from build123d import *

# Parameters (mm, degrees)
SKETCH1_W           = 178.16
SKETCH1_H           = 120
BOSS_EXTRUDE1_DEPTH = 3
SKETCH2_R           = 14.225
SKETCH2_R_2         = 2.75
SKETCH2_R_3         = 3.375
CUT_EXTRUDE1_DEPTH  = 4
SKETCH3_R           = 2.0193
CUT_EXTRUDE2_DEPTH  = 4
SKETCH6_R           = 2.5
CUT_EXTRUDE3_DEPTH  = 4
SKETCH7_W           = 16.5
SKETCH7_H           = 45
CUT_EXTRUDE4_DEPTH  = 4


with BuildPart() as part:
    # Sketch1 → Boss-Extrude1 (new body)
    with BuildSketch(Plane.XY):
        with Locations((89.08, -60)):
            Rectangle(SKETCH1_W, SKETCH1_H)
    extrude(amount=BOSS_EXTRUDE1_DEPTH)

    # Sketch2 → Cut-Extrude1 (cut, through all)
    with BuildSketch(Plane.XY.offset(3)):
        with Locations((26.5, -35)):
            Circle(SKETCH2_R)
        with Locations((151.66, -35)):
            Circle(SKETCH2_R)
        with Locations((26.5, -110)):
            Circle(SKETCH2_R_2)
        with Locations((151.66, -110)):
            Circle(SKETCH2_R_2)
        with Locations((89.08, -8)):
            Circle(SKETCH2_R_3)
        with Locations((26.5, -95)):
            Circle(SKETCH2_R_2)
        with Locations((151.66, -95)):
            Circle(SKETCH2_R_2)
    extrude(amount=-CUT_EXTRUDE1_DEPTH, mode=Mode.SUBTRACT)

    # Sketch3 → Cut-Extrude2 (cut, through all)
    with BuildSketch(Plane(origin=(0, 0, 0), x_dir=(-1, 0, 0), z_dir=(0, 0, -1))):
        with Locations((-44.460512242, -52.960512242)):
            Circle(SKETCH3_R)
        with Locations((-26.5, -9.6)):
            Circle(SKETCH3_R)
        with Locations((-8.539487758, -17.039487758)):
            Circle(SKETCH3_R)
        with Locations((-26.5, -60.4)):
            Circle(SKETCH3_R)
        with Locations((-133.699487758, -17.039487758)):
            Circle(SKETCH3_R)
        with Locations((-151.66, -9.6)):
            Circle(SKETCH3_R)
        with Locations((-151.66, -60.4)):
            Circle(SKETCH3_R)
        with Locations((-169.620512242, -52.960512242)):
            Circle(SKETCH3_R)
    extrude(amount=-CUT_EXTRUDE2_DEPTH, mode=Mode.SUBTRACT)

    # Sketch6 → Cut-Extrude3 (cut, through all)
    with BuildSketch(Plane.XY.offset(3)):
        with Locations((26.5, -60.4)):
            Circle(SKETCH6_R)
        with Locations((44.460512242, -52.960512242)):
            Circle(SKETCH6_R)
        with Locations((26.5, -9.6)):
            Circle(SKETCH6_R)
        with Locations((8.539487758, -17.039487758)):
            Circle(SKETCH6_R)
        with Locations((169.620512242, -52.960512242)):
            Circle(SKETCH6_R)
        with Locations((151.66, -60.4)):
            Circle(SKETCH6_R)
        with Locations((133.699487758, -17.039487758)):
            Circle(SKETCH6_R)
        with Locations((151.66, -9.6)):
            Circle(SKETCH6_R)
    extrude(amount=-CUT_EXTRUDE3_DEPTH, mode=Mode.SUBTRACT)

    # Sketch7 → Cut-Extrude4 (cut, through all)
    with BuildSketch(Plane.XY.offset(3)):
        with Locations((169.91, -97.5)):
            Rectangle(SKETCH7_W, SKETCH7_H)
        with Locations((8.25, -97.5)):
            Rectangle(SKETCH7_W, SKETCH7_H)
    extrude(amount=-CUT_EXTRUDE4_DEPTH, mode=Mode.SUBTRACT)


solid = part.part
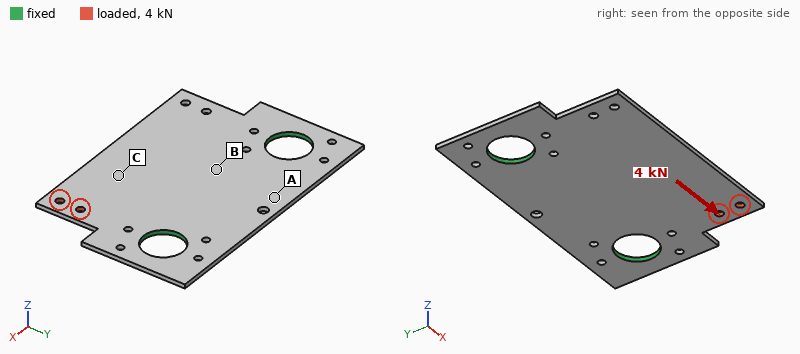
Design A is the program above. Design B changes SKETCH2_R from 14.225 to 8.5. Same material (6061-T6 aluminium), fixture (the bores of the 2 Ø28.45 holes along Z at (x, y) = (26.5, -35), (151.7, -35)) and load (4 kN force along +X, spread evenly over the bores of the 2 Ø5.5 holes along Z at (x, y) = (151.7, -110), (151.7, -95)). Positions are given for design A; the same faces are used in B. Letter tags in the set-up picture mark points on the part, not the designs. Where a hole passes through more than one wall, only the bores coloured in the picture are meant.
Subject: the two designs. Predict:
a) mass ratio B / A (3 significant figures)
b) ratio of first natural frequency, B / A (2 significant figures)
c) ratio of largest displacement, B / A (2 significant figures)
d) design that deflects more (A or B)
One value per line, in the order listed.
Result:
1.04
0.86
1.1
B
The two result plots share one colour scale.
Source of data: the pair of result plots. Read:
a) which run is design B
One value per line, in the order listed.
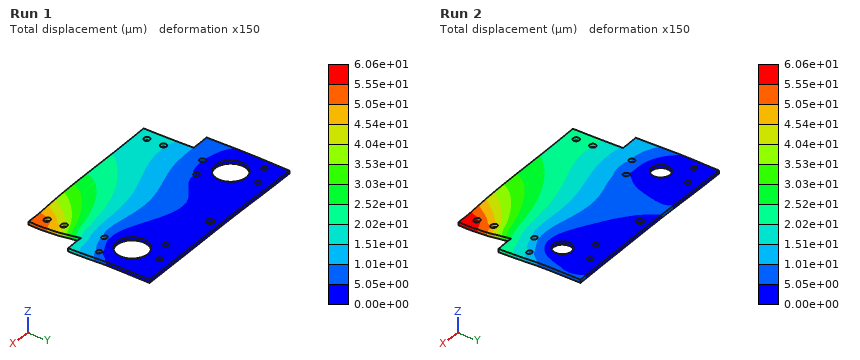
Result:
Run 2
